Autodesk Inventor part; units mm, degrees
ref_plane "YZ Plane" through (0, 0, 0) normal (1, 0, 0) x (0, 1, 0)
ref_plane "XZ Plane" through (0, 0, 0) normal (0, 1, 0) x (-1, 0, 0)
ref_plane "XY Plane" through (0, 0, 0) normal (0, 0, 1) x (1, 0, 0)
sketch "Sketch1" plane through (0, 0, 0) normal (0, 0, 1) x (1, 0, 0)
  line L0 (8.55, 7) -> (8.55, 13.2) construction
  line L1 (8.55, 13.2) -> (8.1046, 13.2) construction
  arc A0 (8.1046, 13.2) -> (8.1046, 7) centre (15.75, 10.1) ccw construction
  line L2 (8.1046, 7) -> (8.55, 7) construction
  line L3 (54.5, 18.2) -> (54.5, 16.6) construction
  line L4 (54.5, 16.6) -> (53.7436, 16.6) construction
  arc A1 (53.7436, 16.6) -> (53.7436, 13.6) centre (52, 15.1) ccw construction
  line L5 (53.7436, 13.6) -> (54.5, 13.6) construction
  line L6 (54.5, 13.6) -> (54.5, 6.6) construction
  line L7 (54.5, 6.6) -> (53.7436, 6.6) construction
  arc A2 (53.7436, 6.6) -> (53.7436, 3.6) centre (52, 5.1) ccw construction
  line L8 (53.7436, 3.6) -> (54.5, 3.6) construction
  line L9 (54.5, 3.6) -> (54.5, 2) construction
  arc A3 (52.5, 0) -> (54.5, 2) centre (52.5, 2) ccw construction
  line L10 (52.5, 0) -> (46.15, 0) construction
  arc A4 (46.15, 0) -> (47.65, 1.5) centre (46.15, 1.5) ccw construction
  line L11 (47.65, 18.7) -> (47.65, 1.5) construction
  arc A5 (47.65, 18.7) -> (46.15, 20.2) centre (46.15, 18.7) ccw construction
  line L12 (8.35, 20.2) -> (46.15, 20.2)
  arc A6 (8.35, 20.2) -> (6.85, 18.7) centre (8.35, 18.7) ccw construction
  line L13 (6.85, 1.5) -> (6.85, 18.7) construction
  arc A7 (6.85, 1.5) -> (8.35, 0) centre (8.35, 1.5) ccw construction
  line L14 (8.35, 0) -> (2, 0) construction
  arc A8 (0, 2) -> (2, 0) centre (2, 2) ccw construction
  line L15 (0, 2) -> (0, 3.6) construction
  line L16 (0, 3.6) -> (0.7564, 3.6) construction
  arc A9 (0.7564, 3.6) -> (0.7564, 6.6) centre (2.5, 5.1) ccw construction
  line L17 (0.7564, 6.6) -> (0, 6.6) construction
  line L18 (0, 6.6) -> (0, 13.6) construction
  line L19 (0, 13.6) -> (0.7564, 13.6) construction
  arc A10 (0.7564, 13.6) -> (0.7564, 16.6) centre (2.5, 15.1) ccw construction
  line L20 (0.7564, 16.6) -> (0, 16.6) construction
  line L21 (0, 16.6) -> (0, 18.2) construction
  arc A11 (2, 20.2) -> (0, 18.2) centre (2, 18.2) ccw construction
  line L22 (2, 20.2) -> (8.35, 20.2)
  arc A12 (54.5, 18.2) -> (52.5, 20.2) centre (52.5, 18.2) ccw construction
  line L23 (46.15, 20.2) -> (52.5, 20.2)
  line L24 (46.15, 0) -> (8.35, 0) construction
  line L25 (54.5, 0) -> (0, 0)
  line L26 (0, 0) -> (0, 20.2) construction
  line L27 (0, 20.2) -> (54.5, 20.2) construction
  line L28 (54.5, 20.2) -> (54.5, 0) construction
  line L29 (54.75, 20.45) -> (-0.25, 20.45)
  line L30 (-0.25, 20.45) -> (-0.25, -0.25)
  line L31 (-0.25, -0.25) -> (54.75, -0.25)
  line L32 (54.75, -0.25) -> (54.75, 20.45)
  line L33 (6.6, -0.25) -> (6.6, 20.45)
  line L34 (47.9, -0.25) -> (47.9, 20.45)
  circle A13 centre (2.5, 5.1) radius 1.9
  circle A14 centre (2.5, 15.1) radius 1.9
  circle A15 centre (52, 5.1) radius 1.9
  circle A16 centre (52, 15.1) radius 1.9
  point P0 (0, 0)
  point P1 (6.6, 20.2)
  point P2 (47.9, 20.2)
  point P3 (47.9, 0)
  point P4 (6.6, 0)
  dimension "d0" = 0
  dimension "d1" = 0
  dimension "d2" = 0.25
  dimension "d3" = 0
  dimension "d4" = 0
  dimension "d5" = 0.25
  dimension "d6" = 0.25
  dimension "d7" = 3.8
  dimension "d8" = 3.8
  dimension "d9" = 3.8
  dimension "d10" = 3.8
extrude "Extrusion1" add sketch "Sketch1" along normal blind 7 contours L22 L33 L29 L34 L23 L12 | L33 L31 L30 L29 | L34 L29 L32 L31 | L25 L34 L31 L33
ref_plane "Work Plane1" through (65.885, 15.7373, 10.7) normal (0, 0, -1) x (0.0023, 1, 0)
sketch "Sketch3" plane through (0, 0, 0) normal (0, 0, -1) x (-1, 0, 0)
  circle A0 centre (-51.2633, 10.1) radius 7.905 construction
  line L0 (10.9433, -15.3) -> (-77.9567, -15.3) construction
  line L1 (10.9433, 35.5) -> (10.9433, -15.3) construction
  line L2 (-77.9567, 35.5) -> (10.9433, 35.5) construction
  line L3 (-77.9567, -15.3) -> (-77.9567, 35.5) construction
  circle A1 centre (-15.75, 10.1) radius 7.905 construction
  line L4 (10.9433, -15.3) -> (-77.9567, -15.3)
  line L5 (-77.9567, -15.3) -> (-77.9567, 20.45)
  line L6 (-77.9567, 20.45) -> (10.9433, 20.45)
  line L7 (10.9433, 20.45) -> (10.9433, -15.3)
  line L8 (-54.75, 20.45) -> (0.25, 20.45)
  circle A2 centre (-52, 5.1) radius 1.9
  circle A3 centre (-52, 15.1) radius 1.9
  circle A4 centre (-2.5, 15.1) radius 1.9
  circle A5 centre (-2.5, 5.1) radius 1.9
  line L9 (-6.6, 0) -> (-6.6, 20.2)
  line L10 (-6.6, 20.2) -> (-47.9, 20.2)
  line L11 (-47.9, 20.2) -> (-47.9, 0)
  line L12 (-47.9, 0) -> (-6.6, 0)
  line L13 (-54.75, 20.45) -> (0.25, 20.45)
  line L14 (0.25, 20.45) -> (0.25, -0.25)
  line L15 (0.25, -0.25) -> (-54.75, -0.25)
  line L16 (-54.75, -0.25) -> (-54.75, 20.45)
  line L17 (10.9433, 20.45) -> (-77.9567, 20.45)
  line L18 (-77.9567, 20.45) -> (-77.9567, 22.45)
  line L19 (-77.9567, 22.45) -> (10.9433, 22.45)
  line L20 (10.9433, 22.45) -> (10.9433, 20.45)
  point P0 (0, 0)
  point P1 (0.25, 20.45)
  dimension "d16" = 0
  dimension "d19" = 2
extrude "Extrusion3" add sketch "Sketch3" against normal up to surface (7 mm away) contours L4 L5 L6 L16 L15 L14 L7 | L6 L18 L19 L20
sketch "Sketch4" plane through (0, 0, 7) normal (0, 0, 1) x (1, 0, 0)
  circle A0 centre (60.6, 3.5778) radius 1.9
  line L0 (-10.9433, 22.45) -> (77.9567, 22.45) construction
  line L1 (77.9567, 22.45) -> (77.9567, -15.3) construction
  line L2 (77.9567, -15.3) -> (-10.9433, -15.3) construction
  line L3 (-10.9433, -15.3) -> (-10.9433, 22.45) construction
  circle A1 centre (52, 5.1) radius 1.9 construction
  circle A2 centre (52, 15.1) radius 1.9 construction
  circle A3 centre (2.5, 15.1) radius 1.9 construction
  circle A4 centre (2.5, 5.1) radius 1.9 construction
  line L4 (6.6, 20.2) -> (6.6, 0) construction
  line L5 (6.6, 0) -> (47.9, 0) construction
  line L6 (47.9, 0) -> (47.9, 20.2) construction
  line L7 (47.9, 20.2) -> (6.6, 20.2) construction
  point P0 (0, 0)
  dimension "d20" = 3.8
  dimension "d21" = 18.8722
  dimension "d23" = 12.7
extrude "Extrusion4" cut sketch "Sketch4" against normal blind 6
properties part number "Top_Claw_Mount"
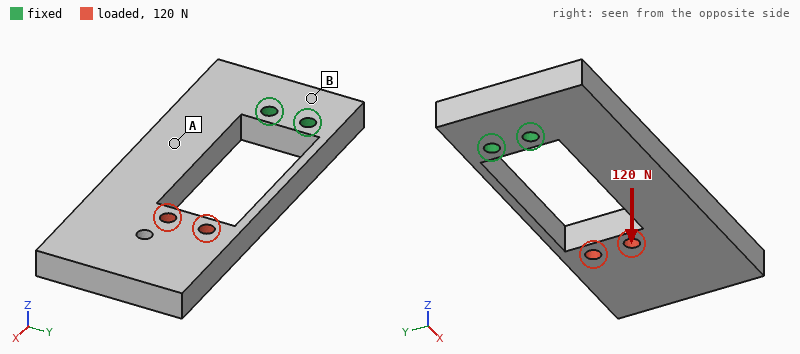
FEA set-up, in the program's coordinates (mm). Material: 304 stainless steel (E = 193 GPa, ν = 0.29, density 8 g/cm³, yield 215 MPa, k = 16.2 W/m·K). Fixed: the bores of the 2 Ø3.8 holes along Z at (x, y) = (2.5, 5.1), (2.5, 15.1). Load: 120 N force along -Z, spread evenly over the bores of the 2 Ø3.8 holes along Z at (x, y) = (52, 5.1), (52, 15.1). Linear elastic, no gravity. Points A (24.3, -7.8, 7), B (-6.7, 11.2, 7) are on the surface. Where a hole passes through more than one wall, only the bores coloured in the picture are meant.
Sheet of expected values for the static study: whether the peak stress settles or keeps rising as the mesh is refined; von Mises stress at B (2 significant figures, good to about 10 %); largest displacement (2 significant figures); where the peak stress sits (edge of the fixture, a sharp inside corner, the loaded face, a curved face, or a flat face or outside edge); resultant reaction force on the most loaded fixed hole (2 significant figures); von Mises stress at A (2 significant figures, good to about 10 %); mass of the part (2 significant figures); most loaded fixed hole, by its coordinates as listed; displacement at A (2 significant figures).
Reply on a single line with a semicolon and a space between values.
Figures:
keeps rising; 7.8 MPa; 0.13 mm; edge of the fixture; 65 N; 23 MPa; 140 g; (2.5, 5.1); 0.021 mm
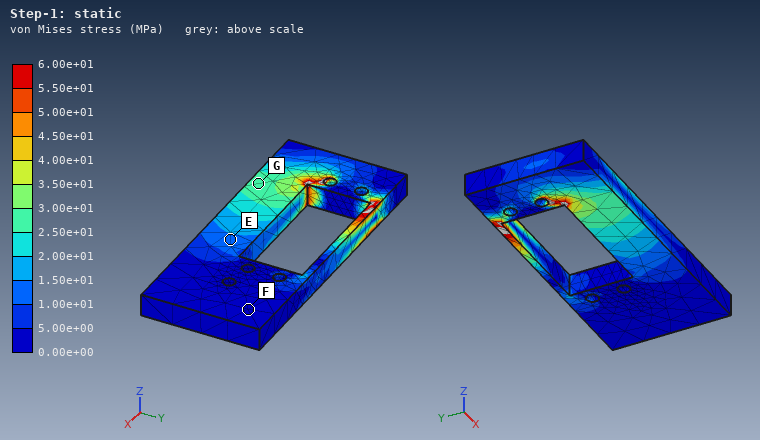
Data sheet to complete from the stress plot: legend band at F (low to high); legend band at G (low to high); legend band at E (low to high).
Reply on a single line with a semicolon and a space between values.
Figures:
0.00e+00 to 5.00e+00 MPa; 2.50e+01 to 3.00e+01 MPa; 1.00e+01 to 1.50e+01 MPa
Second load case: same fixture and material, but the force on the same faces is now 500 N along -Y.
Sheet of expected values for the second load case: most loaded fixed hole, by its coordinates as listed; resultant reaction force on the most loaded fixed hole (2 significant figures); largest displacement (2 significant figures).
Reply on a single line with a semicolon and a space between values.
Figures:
(2.5, 5.1); 1.9 kN; 67 µm
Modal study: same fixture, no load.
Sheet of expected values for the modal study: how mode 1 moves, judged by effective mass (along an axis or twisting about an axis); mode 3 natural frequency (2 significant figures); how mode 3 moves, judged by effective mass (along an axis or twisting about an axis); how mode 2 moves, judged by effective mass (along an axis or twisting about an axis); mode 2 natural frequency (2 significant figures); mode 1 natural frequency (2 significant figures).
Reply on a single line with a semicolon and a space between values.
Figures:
along Z; 2300 Hz; twisting about X; along Y; 1600 Hz; 590 Hz
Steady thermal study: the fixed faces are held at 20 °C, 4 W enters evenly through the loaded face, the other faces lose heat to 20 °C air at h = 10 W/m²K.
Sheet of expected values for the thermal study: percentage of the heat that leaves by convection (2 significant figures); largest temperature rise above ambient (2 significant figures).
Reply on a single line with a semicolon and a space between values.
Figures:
62 %; 69 K
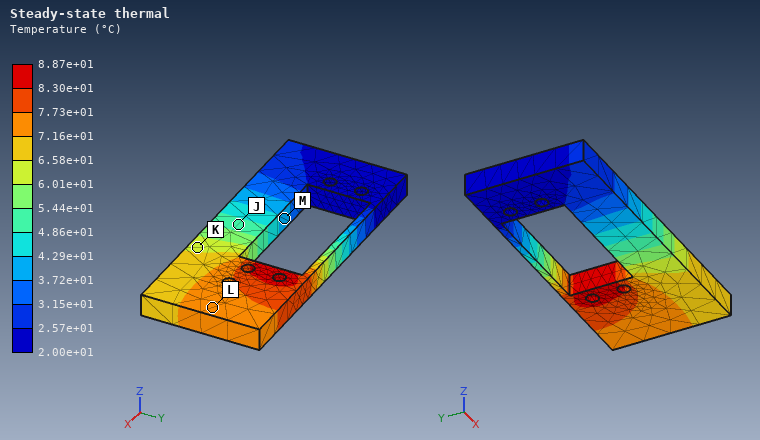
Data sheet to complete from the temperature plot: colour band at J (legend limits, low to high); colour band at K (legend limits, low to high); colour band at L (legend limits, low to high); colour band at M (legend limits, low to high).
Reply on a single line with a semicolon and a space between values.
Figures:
4.86e+01 to 5.44e+01 °C; 6.01e+01 to 6.58e+01 °C; 7.16e+01 to 7.73e+01 °C; 3.72e+01 to 4.29e+01 °C
